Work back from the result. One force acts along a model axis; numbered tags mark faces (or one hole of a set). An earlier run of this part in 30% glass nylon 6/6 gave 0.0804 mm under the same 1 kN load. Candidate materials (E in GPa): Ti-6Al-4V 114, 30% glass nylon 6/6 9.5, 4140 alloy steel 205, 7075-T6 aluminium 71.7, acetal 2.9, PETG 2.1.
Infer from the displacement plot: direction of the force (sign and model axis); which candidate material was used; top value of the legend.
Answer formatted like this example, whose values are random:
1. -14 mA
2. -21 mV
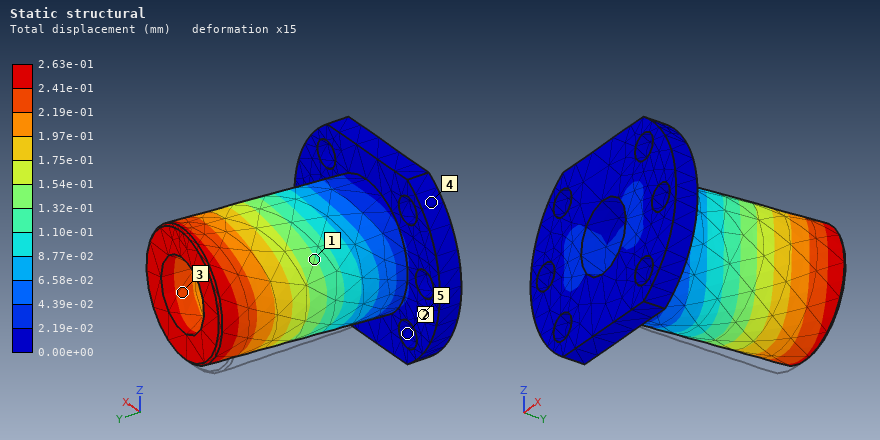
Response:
1. +X
2. acetal
3. 2.63e-01 mm
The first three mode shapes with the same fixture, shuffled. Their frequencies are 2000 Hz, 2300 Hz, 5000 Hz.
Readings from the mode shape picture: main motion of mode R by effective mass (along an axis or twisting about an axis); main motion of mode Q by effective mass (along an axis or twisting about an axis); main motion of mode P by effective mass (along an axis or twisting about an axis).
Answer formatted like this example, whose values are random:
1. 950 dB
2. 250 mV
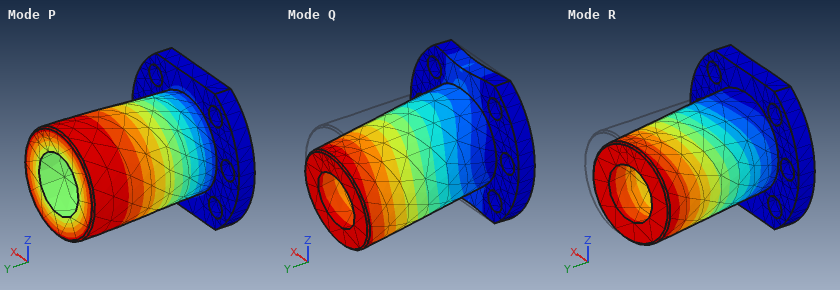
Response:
1. along X
2. along Z
3. twisting about Y
